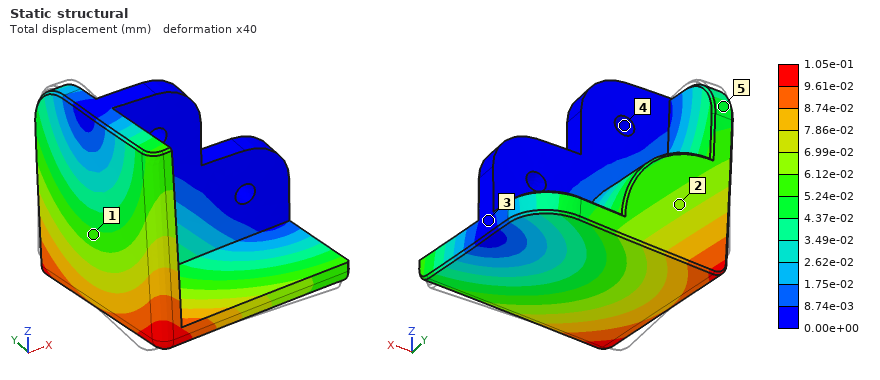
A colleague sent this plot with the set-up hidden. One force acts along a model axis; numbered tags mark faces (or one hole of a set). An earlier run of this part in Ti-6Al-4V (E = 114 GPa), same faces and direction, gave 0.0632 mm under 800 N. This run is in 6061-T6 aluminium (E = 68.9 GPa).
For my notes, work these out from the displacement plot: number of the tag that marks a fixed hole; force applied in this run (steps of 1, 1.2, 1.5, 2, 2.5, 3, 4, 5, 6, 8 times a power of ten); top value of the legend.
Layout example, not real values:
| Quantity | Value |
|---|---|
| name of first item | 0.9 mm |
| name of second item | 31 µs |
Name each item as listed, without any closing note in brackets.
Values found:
| Quantity | Value |
|---|---|
| number of the tag that marks a fixed hole | 4 |
| force applied in this run | 800 N |
| top value of the legend | 1.05e-01 mm |
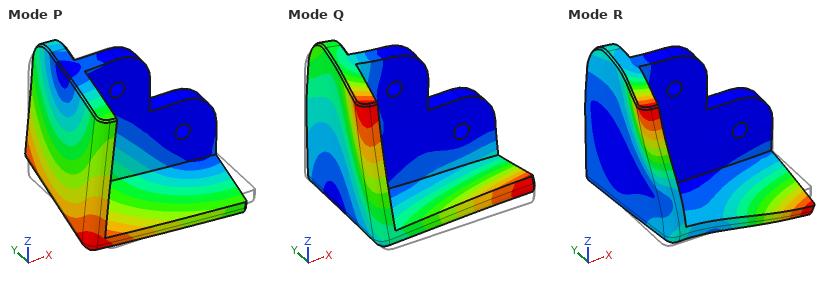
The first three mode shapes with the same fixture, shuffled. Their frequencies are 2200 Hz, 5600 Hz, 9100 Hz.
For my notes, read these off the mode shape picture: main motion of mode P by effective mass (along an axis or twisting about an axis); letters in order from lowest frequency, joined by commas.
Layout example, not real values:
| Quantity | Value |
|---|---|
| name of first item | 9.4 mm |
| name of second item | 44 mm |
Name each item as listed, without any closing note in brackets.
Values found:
| Quantity | Value |
|---|---|
| main motion of mode P by effective mass | along Y |
| letters in order from lowest frequency, joined by commas | P, Q, R |
